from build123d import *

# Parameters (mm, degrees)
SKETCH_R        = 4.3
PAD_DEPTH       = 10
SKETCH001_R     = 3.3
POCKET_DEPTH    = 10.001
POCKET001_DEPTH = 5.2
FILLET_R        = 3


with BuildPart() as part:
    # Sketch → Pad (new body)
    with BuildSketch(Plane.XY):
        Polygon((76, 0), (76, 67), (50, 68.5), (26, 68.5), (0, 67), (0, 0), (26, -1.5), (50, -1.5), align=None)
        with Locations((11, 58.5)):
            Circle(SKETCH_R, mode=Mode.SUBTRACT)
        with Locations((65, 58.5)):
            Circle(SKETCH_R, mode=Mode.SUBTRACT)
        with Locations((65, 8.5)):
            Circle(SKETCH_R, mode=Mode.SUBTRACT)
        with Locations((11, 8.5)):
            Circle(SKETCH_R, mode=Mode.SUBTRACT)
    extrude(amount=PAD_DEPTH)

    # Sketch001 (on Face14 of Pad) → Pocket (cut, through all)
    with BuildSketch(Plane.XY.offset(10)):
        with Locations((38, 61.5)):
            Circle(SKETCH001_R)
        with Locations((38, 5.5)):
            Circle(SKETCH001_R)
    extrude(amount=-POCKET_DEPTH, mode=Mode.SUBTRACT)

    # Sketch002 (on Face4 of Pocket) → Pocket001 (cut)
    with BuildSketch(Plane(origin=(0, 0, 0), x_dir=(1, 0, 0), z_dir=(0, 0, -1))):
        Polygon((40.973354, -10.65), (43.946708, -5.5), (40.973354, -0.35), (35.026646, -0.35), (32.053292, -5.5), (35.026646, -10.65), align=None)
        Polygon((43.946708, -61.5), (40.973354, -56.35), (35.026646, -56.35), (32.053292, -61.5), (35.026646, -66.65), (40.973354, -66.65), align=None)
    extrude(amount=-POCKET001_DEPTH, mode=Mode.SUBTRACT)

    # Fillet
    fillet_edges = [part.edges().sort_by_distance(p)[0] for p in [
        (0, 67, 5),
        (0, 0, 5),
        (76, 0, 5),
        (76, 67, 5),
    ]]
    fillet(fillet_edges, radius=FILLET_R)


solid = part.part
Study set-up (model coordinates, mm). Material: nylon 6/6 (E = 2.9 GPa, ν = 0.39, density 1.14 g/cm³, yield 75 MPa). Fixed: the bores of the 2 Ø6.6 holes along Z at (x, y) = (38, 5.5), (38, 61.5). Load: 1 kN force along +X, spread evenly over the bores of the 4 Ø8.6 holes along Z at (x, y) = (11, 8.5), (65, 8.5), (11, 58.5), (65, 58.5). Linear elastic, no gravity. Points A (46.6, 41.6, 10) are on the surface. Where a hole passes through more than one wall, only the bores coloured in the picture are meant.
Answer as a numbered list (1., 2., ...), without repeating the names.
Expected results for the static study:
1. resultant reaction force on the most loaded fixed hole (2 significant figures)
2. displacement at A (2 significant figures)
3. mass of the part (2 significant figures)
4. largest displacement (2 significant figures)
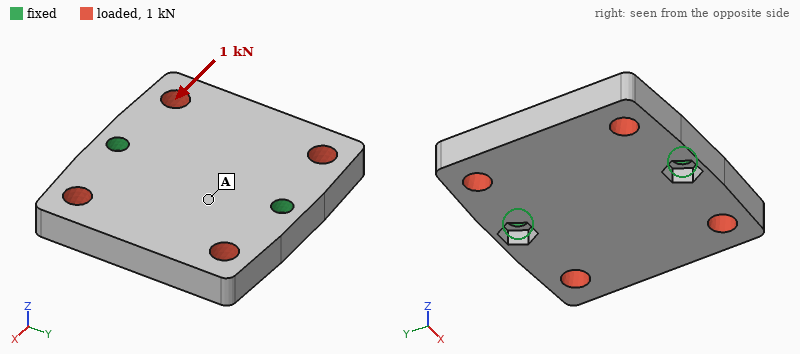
1. 500 N
2. 0.031 mm
3. 56 g
4. 0.15 mm
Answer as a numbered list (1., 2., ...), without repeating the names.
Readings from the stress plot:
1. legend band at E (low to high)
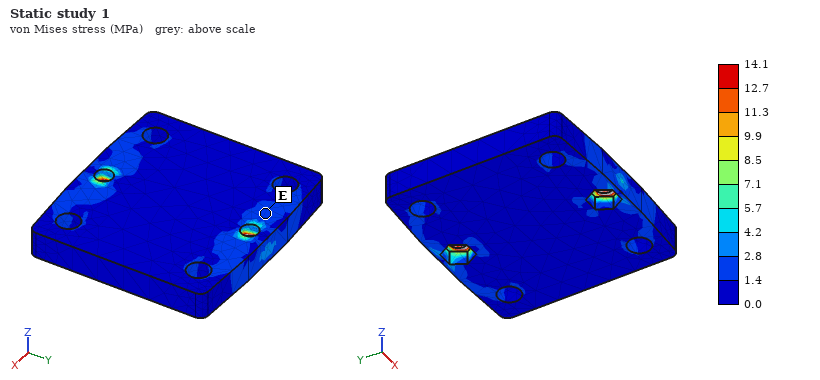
1. 1.4 to 2.8 MPa
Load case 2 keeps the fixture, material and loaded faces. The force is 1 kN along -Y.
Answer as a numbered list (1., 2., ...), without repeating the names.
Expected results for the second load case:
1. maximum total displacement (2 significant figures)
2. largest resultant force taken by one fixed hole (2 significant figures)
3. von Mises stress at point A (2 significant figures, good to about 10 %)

1. 47 µm
2. 500 N
3. 1.5 MPa
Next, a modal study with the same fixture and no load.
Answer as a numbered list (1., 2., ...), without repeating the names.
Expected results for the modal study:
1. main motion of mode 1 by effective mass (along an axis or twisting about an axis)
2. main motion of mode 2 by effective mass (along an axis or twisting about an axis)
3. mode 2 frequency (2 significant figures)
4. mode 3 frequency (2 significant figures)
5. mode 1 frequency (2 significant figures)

1. twisting about Y
2. along Z
3. 1500 Hz
4. 2200 Hz
5. 780 Hz
